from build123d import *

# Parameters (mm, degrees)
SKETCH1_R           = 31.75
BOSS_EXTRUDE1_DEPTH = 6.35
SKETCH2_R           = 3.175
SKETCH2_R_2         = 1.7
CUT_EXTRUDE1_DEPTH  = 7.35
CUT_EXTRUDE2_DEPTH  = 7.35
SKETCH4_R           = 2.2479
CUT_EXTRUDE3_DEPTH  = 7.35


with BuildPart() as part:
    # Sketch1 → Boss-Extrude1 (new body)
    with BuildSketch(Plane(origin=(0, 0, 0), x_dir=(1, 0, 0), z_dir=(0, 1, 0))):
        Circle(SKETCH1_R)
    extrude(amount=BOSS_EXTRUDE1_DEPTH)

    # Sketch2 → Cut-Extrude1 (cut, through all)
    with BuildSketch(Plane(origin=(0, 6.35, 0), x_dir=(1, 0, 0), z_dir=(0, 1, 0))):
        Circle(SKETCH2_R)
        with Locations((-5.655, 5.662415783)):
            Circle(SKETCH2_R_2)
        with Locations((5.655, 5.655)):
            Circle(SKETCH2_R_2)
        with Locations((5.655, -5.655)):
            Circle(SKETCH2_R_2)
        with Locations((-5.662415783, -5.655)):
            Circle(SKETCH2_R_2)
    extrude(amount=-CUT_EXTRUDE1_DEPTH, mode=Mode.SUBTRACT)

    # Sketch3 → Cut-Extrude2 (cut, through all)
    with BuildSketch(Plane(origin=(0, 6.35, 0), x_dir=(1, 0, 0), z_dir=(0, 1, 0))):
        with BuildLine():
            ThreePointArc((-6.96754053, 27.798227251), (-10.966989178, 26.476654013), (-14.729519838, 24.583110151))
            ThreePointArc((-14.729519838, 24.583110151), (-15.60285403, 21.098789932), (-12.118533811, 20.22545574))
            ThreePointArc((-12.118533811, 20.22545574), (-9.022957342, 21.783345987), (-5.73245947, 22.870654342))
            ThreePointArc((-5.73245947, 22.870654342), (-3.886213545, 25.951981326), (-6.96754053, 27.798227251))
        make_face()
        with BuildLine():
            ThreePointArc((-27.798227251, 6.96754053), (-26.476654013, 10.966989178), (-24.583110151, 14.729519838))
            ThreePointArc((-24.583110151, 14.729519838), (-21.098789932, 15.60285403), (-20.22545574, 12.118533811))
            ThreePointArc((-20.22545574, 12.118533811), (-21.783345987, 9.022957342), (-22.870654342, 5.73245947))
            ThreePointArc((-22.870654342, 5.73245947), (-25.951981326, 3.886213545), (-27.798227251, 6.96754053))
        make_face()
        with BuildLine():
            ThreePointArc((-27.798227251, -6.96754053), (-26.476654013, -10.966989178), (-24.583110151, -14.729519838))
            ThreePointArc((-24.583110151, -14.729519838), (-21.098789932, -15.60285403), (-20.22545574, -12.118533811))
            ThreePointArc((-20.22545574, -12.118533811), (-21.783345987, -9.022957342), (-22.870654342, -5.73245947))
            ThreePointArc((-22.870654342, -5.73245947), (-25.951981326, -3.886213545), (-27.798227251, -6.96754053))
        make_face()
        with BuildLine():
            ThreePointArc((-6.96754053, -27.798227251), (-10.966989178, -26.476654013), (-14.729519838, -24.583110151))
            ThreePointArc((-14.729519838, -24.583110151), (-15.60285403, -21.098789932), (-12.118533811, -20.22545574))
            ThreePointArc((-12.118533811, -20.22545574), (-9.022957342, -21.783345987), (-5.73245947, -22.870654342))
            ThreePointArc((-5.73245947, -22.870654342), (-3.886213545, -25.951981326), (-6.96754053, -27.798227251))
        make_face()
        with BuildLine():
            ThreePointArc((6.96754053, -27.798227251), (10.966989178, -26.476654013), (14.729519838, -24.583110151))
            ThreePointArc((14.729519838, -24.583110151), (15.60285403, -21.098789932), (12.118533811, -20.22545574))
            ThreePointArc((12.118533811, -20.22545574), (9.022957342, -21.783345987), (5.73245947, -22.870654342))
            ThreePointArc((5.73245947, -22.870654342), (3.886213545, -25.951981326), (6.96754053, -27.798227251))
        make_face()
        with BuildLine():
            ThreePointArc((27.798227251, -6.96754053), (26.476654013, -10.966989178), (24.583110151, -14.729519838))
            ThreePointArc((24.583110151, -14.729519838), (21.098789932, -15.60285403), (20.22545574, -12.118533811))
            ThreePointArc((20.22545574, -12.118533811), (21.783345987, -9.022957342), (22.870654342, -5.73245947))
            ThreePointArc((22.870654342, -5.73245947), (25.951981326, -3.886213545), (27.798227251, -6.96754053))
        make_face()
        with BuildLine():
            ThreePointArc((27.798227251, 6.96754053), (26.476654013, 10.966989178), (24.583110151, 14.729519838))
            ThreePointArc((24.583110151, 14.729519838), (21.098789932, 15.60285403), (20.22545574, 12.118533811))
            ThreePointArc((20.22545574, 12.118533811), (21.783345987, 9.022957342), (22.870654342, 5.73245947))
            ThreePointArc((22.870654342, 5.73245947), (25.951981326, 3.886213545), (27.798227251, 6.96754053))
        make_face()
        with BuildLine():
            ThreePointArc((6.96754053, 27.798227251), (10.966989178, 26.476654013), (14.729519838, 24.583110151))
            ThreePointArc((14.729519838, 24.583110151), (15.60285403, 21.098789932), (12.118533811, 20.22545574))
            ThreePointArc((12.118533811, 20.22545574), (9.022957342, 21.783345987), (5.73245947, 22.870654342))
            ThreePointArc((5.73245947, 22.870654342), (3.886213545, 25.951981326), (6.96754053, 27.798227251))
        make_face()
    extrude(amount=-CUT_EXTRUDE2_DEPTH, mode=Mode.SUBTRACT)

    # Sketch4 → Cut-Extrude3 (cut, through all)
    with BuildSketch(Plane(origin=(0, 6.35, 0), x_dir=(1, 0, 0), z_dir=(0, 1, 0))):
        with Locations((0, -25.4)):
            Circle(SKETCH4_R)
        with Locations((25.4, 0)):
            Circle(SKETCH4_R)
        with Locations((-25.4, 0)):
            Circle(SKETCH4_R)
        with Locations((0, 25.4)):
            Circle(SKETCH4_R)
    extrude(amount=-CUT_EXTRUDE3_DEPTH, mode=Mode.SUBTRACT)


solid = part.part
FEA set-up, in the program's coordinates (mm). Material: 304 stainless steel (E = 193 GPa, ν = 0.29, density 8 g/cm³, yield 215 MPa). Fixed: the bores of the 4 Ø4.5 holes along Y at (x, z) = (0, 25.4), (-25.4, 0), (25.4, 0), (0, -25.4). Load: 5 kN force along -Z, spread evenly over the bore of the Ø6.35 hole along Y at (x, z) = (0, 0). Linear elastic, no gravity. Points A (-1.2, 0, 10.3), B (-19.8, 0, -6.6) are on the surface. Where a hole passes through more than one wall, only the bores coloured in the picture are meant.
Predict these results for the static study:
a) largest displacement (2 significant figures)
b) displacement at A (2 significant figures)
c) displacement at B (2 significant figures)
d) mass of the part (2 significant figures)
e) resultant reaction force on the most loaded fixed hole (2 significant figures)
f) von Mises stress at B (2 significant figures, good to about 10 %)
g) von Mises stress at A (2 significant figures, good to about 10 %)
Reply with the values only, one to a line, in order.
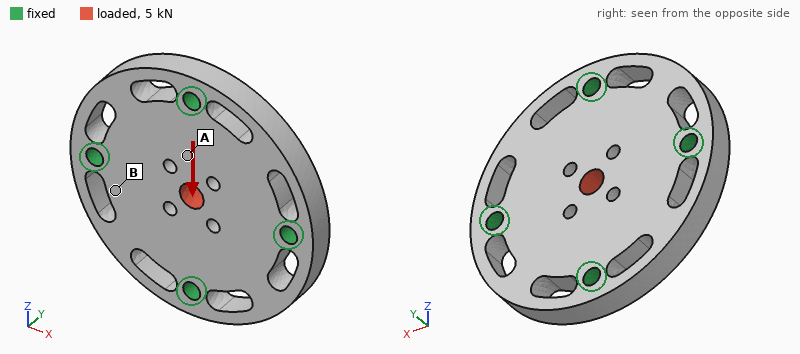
3.6 µm
2.0 µm
0.89 µm
130 g
1.8 kN
7.4 MPa
32 MPa
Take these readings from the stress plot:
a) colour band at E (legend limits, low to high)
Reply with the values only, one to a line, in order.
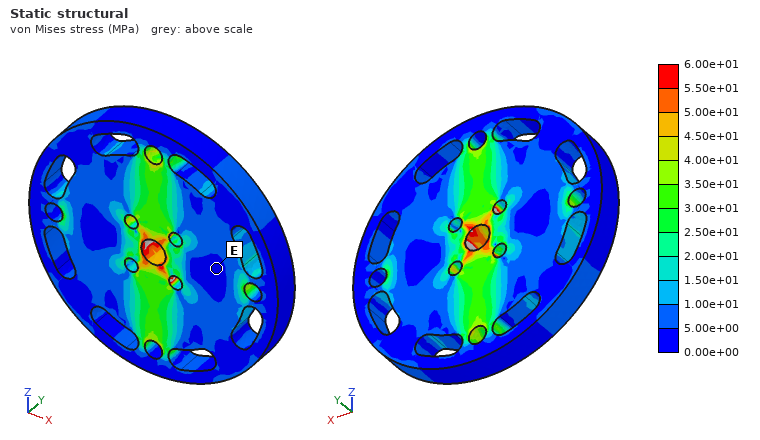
0.00e+00 to 5.00e+00 MPa
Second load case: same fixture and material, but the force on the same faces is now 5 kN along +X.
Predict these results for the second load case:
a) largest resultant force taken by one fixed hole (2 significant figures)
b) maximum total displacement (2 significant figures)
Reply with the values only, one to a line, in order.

1.8 kN
3.6 µm
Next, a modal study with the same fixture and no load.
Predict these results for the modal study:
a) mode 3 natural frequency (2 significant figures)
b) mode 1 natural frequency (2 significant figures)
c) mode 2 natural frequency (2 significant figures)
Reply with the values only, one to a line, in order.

15 kHz
15 kHz
15 kHz
